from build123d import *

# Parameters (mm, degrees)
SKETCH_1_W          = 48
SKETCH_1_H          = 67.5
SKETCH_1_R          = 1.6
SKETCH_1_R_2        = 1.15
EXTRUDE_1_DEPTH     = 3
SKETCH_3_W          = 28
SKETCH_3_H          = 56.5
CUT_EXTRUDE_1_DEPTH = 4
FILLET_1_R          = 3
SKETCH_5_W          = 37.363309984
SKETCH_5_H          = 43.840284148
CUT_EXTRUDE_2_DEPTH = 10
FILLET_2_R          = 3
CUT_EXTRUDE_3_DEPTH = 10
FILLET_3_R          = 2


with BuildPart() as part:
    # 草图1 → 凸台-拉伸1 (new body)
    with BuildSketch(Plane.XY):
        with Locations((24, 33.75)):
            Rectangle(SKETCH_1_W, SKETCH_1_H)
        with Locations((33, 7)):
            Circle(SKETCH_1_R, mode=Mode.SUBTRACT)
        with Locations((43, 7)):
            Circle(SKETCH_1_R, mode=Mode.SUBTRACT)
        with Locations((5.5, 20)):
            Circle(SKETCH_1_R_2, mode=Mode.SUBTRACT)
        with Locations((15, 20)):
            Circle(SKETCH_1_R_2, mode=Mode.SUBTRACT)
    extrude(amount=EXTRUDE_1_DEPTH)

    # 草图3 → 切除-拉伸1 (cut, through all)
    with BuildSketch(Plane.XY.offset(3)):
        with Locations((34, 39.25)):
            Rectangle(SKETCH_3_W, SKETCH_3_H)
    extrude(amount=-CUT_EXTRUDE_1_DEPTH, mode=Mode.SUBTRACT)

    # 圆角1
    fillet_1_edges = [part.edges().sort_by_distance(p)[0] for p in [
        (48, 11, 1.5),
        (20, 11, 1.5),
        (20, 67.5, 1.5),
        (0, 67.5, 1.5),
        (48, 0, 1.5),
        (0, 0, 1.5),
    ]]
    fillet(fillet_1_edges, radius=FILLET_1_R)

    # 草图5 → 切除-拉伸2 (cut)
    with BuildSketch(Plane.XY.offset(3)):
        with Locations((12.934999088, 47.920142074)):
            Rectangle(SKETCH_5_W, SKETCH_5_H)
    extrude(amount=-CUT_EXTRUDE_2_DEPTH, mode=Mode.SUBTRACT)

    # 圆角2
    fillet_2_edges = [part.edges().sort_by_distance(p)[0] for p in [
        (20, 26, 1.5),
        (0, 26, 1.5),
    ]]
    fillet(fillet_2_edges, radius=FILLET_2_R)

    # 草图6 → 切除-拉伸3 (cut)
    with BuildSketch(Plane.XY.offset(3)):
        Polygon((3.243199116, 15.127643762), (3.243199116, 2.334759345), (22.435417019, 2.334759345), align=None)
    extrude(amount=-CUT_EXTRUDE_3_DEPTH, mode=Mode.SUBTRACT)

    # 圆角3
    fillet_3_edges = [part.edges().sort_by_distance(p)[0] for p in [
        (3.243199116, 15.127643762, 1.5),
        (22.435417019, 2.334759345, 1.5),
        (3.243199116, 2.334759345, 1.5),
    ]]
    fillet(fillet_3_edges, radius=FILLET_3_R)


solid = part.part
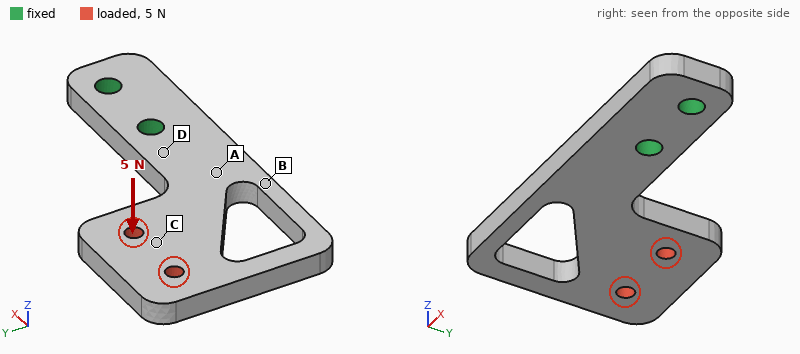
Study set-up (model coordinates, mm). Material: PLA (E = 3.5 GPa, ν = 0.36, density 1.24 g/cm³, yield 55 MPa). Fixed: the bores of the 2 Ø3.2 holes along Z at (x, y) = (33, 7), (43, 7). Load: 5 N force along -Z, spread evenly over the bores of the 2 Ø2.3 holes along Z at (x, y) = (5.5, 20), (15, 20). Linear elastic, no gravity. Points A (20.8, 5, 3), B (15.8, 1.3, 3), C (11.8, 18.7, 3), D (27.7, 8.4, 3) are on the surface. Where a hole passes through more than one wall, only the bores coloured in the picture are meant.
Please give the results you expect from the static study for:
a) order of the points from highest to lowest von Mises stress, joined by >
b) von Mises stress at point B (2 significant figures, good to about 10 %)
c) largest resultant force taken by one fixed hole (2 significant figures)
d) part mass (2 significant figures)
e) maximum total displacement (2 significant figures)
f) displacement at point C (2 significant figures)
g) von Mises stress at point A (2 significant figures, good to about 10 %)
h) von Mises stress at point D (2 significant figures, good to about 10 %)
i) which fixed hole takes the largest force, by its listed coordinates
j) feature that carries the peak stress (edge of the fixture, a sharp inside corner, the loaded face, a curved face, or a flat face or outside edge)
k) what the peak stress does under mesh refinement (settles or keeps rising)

D > A > B > C
2.6 MPa
6.3 N
2.5 g
0.62 mm
0.35 mm
4.7 MPa
7.0 MPa
(33, 7)
edge of the fixture
keeps rising
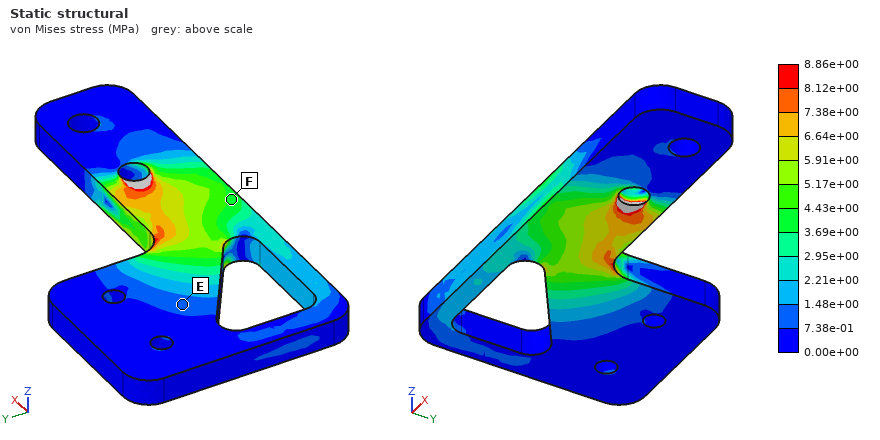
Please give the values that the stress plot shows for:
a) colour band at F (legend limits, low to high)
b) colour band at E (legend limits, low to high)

3.69e+00 to 4.43e+00 MPa
7.38e-01 to 1.48e+00 MPa
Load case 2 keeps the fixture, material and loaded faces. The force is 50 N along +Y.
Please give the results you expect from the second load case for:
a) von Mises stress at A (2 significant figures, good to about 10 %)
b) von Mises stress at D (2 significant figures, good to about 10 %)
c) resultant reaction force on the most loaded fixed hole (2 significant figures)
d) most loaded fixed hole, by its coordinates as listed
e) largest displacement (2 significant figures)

8.7 MPa
7.9 MPa
120 N
(33, 7)
0.62 mm
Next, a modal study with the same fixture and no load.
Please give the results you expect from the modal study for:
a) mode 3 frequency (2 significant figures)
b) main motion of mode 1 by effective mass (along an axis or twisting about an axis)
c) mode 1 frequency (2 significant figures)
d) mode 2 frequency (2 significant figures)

1300 Hz
along Z
520 Hz
1300 Hz
